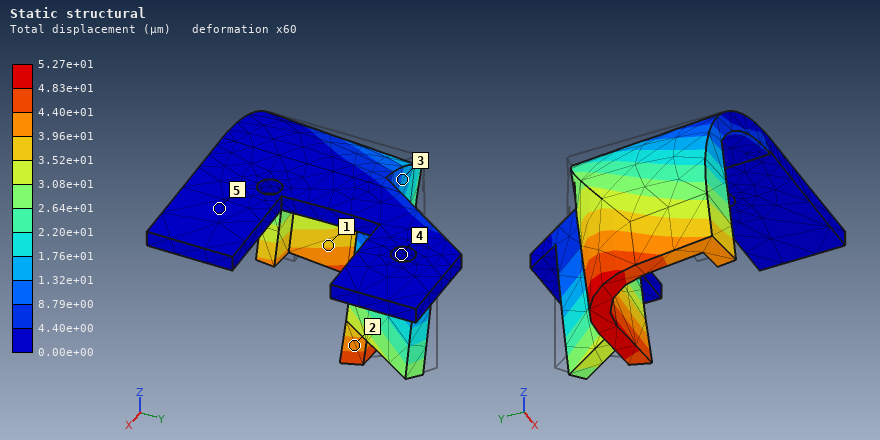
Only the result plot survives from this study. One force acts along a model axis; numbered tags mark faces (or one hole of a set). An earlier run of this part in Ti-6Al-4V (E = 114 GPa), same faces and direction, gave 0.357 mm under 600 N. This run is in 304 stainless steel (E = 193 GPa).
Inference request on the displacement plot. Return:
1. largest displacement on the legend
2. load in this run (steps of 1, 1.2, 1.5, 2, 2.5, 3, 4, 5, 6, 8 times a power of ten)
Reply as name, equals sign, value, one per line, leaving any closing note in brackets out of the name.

largest displacement on the legend = 5.27e+01 µm
load in this run = 150 N
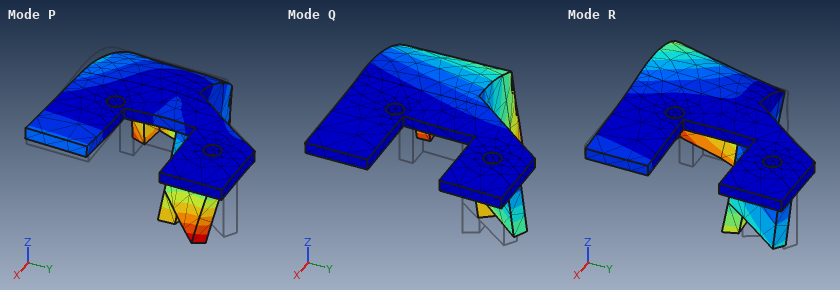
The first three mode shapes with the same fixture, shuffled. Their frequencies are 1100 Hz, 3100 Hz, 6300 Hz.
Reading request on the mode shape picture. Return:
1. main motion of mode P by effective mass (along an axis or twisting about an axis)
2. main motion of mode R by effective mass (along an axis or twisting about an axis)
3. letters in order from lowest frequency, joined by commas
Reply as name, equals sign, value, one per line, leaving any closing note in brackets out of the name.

main motion of mode P by effective mass = twisting about Z
main motion of mode R by effective mass = along Y
letters in order from lowest frequency, joined by commas = Q, R, P
